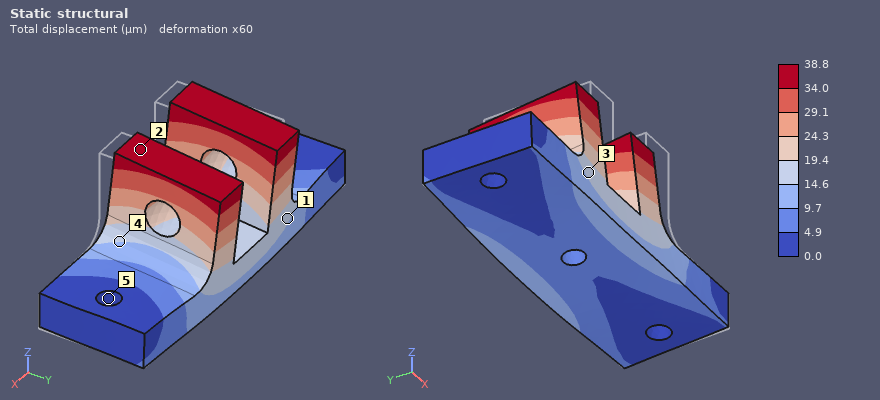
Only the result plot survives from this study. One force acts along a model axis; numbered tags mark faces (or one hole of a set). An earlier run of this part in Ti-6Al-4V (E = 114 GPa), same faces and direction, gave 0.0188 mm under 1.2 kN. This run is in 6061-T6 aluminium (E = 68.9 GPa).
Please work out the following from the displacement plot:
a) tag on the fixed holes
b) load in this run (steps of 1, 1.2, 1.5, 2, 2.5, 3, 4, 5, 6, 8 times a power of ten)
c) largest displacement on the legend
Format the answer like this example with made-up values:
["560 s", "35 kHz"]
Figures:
["5", "1.5 kN", "38.8 µm"]
